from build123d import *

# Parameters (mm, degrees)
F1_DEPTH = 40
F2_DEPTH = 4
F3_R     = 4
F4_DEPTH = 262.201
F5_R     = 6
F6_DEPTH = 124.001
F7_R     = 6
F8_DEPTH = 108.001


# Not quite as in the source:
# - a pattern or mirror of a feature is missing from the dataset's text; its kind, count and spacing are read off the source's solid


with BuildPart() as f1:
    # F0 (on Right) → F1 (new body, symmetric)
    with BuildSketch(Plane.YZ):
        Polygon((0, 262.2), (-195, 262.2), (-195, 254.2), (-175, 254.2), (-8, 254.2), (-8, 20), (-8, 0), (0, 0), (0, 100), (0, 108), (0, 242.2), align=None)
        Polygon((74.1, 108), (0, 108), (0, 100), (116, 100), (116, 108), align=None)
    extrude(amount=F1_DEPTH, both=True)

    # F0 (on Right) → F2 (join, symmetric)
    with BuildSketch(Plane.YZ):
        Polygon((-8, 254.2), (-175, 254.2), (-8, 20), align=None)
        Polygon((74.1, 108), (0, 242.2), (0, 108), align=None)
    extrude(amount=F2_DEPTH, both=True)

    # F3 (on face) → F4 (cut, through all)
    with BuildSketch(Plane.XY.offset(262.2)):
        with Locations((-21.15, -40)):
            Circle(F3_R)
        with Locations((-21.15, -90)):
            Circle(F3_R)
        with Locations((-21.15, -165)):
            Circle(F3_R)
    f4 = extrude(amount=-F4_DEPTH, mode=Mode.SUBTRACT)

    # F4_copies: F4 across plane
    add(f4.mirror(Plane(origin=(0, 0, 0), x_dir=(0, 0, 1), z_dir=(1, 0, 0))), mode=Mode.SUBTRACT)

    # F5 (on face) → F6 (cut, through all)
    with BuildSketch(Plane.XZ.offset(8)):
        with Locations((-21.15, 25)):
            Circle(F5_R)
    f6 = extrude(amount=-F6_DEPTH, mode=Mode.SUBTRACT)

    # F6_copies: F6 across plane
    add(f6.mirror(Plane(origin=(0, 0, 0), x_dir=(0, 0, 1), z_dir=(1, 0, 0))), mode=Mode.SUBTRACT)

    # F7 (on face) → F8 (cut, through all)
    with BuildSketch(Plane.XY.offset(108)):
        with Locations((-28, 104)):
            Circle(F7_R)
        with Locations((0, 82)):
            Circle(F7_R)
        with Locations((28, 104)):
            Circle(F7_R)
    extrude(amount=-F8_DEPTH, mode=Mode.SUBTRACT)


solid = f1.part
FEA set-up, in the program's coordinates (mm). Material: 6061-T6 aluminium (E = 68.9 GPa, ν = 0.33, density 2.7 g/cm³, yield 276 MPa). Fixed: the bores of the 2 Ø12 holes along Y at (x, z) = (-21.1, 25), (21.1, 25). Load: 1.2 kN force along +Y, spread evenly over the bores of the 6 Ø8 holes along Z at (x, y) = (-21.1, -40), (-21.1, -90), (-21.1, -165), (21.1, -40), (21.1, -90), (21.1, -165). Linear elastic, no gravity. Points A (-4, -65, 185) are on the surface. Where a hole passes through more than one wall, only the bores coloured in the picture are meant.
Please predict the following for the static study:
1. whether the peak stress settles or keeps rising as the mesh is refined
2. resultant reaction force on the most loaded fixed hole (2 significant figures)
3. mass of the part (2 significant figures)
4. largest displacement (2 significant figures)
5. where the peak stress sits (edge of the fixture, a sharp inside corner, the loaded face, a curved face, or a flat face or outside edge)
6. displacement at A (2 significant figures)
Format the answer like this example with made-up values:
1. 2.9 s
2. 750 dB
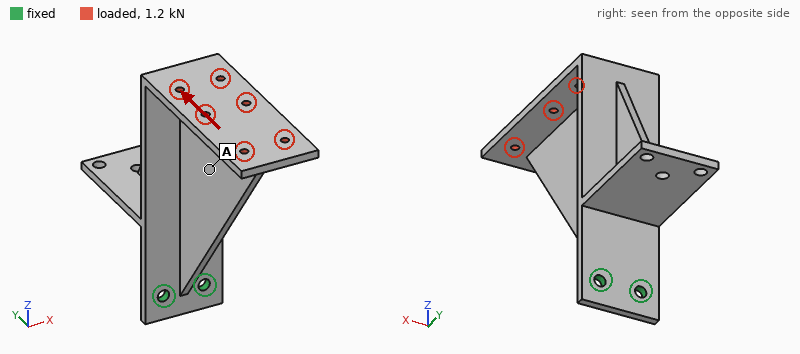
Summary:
1. keeps rising
2. 910 N
3. 1.5 kg
4. 4.8 mm
5. edge of the fixture
6. 2.6 mm
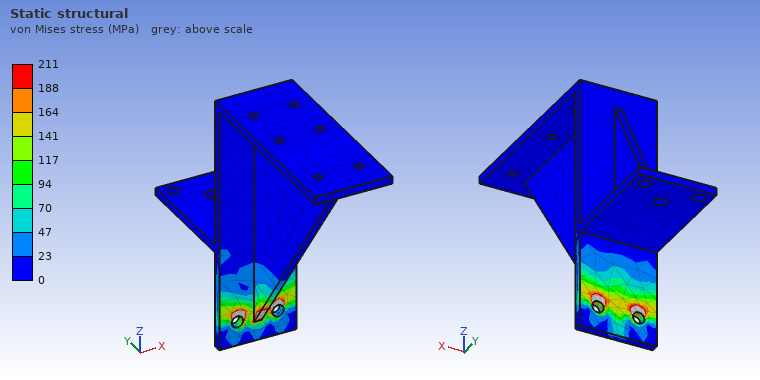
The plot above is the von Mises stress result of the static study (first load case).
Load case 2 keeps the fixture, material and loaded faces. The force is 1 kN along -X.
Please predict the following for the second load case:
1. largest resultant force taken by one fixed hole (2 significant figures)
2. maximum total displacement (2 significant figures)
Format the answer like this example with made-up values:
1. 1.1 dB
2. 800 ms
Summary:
1. 5.2 kN
2. 4.6 mm
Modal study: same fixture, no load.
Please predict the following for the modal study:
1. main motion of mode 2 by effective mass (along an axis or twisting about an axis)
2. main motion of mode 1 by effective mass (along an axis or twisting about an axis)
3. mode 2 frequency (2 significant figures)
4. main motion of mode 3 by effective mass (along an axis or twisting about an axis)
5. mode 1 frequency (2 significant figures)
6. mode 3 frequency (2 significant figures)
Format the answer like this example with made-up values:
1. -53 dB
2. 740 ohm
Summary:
1. along X
2. along Y
3. 130 Hz
4. along X
5. 100 Hz
6. 530 Hz
